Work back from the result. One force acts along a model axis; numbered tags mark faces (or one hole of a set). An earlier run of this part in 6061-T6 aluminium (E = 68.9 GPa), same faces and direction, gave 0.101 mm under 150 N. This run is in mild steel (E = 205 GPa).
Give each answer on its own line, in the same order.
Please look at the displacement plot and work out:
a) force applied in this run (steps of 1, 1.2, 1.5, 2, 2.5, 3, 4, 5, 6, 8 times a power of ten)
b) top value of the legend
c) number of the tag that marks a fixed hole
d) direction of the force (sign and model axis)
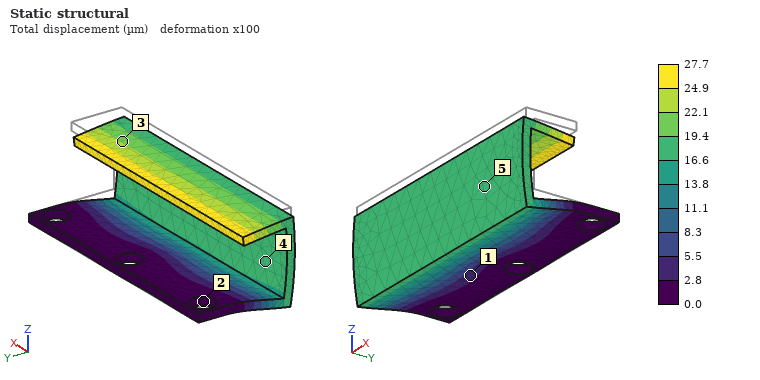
120 N
27.7 µm
2
-Z
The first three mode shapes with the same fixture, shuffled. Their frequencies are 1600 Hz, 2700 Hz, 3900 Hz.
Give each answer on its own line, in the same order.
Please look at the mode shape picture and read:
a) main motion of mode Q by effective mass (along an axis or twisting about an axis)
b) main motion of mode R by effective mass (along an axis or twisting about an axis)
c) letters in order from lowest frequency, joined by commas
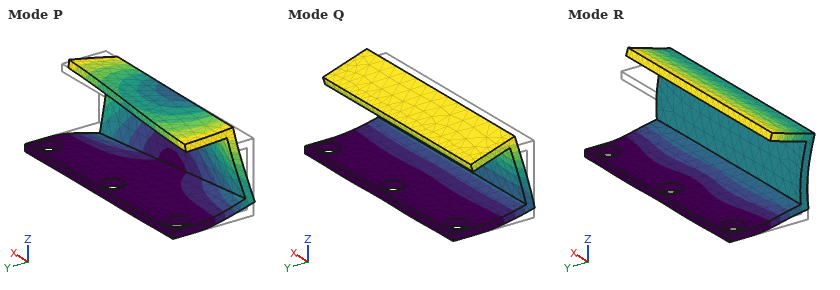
along Y
along Z
Q, P, R
